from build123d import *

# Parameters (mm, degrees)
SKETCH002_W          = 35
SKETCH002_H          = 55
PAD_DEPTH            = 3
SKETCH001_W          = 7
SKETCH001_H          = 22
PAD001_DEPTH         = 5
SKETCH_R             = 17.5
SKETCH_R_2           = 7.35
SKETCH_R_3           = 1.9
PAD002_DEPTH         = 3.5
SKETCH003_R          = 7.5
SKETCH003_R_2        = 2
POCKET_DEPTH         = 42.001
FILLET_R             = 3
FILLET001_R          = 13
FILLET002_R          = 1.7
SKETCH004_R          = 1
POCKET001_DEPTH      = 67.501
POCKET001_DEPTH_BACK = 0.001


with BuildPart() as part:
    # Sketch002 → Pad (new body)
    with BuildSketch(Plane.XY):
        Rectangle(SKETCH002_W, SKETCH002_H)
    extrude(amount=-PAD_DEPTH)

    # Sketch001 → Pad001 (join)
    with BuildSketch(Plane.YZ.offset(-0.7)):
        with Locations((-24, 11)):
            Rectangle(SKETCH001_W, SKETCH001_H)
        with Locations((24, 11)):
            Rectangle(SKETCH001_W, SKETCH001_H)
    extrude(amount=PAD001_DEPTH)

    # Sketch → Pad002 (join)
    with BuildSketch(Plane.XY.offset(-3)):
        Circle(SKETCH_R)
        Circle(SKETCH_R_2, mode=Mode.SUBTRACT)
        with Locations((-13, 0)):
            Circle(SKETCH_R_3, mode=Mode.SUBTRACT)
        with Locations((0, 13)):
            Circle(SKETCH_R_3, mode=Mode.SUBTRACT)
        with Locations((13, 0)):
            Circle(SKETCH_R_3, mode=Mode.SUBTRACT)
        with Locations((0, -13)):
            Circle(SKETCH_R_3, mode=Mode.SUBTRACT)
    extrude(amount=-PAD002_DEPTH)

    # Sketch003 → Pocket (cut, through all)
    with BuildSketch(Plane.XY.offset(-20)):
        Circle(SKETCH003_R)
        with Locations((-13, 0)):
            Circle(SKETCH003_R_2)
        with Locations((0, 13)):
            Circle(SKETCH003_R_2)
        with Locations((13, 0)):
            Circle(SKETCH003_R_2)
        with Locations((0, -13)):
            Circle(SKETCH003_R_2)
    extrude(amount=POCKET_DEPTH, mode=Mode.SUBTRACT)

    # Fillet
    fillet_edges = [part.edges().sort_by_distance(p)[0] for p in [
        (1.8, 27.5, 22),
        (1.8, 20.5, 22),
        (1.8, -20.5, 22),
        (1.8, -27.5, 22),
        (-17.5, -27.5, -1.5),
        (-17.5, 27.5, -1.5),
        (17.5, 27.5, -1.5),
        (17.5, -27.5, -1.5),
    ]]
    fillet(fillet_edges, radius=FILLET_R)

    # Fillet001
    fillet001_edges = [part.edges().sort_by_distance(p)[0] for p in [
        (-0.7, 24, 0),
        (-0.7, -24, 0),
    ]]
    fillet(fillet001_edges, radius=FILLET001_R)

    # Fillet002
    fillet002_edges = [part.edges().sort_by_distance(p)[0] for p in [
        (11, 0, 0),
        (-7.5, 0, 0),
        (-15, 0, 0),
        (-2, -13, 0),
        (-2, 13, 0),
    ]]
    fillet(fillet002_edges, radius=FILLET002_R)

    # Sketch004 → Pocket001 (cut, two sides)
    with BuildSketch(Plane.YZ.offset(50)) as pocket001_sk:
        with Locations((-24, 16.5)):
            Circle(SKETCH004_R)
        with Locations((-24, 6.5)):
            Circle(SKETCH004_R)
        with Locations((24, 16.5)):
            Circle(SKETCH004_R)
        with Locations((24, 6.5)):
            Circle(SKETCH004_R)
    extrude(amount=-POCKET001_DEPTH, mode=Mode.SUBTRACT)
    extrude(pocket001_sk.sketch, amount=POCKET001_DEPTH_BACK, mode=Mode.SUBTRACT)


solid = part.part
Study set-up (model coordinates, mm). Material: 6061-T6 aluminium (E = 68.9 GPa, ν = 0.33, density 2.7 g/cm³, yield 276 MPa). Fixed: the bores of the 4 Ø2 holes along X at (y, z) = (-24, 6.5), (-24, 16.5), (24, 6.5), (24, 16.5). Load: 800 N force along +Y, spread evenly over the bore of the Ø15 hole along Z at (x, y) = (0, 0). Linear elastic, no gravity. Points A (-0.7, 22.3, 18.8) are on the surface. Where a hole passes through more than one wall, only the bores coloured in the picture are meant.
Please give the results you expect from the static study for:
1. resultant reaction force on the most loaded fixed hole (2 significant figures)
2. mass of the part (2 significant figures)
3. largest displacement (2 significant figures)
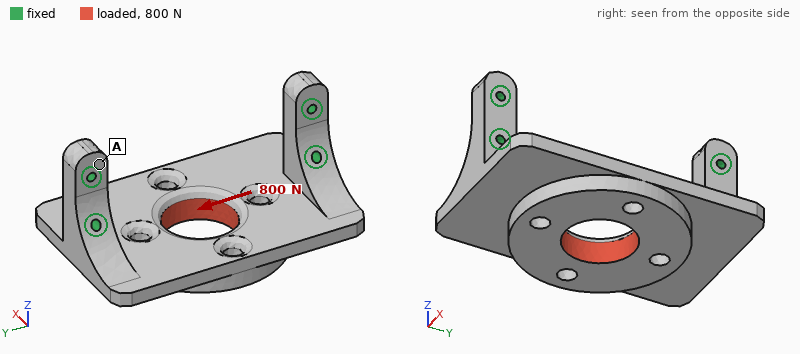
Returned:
510 N
26 g
9.9 µm
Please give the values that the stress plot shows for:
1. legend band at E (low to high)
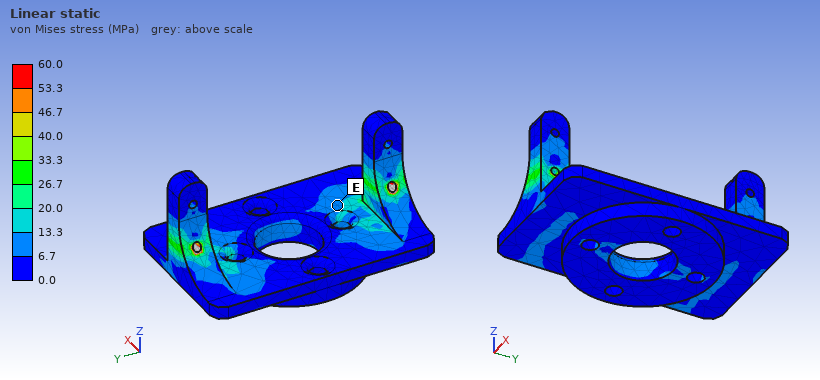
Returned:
6.7 to 13.3 MPa
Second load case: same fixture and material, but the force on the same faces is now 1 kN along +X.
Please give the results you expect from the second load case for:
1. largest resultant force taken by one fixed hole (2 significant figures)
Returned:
550 N
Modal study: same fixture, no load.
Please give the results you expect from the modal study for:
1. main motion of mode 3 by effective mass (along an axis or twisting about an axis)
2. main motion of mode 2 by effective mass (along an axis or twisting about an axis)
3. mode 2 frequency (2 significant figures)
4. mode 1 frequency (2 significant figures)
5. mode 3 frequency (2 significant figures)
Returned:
along Y
along Z
7800 Hz
4900 Hz
9800 Hz
